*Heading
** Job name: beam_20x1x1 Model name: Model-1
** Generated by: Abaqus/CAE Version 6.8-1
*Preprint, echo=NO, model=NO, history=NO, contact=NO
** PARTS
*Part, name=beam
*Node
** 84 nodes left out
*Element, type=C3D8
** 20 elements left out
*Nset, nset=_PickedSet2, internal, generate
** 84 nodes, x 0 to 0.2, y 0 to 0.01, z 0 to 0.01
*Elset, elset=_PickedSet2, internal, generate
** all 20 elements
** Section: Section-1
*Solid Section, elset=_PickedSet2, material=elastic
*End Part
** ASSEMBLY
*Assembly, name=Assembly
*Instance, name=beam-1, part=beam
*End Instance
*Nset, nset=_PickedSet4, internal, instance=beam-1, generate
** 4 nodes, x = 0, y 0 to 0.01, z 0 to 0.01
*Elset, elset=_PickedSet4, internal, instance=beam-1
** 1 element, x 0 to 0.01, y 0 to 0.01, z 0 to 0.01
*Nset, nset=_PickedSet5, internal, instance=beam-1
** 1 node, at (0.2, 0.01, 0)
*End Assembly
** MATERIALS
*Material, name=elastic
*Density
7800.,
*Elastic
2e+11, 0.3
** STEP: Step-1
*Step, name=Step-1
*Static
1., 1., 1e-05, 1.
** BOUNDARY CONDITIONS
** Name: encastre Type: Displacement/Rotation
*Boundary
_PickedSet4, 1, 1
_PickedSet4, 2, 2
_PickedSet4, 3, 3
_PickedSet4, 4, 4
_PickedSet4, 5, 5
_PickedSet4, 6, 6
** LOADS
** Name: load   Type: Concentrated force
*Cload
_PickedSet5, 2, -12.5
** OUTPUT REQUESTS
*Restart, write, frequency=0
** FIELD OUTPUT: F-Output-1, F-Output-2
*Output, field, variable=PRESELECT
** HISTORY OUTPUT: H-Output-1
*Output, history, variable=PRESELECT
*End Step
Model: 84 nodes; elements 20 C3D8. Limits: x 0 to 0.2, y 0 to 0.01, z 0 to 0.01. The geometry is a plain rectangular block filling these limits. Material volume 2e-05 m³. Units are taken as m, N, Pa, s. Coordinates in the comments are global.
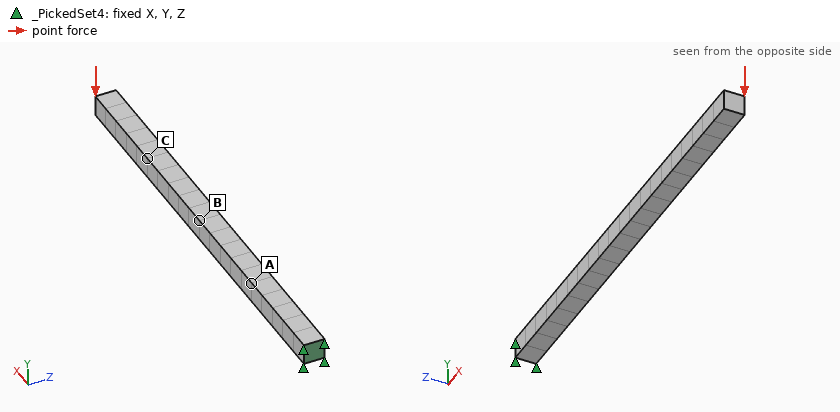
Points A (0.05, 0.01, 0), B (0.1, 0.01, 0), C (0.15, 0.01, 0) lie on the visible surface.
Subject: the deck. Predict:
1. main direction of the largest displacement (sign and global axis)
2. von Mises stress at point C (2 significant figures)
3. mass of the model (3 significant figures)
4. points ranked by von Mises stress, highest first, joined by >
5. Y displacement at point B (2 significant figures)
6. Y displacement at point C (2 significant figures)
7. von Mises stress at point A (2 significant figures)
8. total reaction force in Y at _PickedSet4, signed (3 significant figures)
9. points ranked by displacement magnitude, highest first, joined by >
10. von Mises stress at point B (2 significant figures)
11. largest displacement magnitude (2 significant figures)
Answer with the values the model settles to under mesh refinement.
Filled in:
-Y
3.8e+06 Pa
0.156 kg
A > B > C
-6.2e-05 m
-1.3e-04 m
1.1e+07 Pa
12.5 N
C > B > A
7.5e+06 Pa
2.0e-04 m
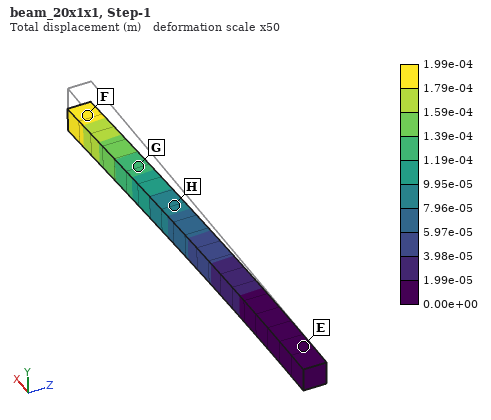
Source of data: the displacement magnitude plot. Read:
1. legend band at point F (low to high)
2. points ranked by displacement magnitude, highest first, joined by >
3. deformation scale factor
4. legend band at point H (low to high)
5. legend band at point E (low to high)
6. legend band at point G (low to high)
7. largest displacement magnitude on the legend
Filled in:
1.79e-04 to 1.99e-04 m
F > G > H > E
50
7.96e-05 to 9.95e-05 m
0.00e+00 to 1.99e-05 m
1.19e-04 to 1.39e-04 m
1.99e-04 m
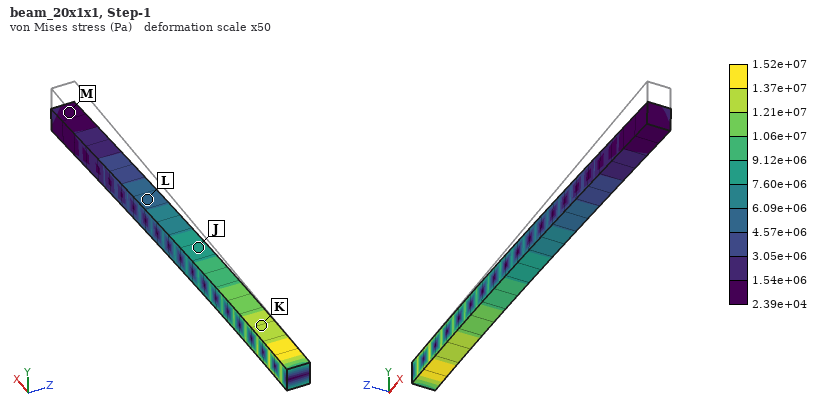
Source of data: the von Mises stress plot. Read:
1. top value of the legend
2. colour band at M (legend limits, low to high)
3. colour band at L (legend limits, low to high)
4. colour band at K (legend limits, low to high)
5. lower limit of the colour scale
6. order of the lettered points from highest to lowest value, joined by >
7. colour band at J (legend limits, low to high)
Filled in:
1.52e+07 Pa
2.39e+04 to 1.54e+06 Pa
4.57e+06 to 6.09e+06 Pa
1.21e+07 to 1.37e+07 Pa
2.39e+04 Pa
K > J > L > M
7.60e+06 to 9.12e+06 Pa
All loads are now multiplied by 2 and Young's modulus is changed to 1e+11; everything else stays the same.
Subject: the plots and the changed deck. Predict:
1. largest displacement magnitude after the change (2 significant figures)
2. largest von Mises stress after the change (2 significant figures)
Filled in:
8.0e-04 m
3.0e+07 Pa
